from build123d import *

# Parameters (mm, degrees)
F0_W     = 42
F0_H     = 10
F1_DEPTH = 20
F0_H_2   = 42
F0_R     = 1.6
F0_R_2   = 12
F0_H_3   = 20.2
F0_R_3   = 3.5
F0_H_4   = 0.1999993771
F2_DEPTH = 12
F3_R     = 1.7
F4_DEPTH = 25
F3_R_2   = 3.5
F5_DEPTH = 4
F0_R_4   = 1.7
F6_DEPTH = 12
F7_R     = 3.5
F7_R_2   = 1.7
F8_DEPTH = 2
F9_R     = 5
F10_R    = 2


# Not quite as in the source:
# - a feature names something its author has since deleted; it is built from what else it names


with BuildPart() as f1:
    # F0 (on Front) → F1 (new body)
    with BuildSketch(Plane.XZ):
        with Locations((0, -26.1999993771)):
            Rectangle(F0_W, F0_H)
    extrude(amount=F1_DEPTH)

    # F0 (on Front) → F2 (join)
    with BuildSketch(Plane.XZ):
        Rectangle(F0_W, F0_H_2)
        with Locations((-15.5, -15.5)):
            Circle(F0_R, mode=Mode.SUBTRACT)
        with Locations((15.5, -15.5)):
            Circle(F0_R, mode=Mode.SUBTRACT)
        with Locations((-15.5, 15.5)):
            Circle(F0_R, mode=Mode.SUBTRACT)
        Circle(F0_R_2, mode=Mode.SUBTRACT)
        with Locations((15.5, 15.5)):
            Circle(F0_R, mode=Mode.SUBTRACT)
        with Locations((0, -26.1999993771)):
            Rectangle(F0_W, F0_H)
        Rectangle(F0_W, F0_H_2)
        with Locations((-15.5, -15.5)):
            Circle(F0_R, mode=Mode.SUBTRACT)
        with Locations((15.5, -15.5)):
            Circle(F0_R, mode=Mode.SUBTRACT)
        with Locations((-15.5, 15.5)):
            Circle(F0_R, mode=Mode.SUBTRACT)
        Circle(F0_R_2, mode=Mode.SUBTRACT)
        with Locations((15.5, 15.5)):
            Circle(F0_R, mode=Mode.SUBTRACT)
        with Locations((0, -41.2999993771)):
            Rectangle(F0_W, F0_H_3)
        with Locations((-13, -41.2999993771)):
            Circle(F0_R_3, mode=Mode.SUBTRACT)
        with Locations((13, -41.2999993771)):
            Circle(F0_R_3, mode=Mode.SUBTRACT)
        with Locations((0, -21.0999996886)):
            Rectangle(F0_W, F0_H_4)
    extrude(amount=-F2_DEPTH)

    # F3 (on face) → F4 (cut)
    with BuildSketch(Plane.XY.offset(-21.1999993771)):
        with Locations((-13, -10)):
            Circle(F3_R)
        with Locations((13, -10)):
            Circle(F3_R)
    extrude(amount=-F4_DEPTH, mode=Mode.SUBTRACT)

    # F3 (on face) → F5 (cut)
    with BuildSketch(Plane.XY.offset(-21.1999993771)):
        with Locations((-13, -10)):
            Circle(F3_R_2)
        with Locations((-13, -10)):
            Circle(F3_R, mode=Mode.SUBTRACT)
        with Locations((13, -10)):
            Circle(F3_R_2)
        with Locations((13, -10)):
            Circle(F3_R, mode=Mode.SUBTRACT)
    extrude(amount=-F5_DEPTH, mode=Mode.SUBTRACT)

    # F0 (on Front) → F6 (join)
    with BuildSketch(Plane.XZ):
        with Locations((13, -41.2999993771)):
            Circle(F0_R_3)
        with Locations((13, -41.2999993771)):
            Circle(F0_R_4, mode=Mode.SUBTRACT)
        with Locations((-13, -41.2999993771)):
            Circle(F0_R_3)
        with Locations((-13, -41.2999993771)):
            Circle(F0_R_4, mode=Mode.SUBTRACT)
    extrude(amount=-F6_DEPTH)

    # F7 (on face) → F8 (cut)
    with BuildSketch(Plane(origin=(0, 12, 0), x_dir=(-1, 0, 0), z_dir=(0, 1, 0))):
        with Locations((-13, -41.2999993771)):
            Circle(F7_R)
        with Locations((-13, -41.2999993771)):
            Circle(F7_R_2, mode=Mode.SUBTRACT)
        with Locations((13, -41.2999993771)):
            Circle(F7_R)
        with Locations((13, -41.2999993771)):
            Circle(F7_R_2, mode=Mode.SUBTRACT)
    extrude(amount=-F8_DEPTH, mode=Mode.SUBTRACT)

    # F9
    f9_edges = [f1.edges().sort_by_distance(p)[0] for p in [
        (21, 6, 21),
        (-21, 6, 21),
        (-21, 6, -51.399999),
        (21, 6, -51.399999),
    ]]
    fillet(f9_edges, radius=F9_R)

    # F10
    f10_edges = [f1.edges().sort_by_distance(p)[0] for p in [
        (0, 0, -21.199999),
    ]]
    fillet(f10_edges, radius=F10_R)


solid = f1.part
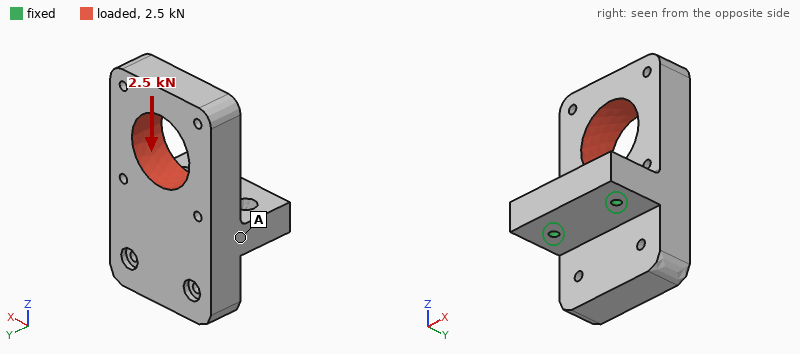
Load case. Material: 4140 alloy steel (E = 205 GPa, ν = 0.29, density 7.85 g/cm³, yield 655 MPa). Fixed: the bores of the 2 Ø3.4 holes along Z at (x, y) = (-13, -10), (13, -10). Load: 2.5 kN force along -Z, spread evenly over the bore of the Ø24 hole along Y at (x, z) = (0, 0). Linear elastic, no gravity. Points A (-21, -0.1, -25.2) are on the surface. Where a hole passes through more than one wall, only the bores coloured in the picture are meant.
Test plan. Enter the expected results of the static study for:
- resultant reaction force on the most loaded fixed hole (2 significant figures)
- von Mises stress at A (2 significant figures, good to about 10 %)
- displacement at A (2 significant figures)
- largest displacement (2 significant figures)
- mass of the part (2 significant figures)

1.3 kN
23 MPa
11 µm
68 µm
300 g
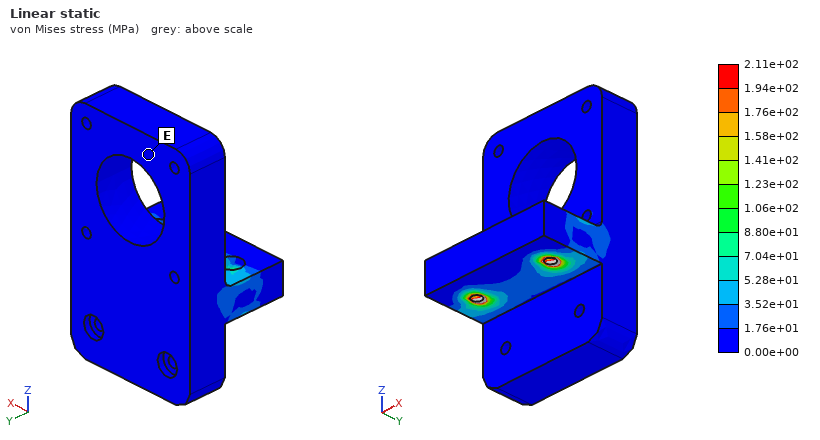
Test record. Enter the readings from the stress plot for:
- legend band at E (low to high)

0.00e+00 to 1.76e+01 MPa
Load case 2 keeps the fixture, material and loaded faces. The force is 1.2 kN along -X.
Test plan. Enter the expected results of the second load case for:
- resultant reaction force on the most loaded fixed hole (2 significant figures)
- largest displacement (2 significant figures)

1.5 kN
16 µm
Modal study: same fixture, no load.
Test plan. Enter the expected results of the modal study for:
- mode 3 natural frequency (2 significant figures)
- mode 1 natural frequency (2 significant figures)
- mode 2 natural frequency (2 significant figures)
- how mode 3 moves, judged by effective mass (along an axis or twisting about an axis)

6400 Hz
1800 Hz
4300 Hz
along Z
